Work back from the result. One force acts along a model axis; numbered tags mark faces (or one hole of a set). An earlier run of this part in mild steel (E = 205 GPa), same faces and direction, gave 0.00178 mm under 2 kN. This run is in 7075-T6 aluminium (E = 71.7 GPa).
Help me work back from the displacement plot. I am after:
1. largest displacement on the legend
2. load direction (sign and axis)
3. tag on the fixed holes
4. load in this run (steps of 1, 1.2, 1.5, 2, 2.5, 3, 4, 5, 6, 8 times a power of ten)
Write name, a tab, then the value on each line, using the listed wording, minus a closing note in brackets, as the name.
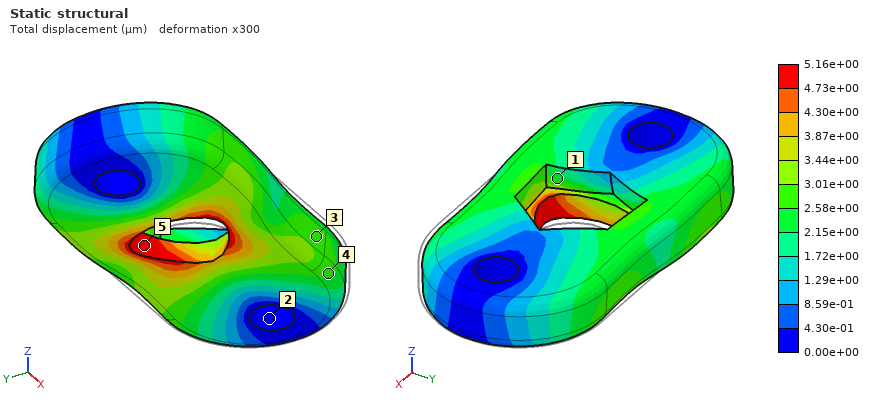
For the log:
largest displacement on the legend	5.16e+00 µm
load direction	-X
tag on the fixed holes	2
load in this run	2 kN
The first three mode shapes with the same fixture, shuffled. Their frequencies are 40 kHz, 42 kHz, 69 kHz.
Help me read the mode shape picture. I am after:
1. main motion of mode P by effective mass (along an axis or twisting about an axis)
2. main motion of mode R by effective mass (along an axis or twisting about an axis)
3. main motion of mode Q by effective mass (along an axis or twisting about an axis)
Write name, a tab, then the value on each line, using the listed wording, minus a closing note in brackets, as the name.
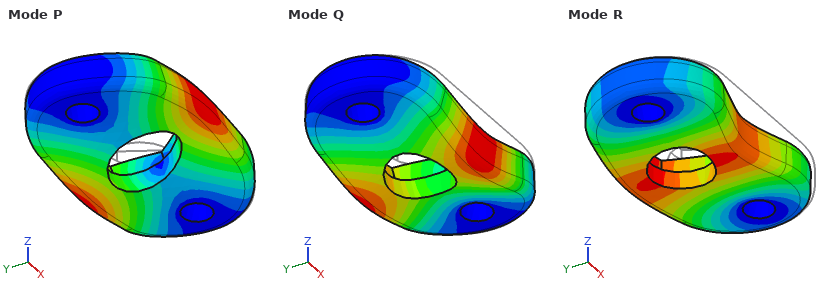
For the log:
main motion of mode P by effective mass	twisting about X
main motion of mode R by effective mass	along Y
main motion of mode Q by effective mass	along Z
